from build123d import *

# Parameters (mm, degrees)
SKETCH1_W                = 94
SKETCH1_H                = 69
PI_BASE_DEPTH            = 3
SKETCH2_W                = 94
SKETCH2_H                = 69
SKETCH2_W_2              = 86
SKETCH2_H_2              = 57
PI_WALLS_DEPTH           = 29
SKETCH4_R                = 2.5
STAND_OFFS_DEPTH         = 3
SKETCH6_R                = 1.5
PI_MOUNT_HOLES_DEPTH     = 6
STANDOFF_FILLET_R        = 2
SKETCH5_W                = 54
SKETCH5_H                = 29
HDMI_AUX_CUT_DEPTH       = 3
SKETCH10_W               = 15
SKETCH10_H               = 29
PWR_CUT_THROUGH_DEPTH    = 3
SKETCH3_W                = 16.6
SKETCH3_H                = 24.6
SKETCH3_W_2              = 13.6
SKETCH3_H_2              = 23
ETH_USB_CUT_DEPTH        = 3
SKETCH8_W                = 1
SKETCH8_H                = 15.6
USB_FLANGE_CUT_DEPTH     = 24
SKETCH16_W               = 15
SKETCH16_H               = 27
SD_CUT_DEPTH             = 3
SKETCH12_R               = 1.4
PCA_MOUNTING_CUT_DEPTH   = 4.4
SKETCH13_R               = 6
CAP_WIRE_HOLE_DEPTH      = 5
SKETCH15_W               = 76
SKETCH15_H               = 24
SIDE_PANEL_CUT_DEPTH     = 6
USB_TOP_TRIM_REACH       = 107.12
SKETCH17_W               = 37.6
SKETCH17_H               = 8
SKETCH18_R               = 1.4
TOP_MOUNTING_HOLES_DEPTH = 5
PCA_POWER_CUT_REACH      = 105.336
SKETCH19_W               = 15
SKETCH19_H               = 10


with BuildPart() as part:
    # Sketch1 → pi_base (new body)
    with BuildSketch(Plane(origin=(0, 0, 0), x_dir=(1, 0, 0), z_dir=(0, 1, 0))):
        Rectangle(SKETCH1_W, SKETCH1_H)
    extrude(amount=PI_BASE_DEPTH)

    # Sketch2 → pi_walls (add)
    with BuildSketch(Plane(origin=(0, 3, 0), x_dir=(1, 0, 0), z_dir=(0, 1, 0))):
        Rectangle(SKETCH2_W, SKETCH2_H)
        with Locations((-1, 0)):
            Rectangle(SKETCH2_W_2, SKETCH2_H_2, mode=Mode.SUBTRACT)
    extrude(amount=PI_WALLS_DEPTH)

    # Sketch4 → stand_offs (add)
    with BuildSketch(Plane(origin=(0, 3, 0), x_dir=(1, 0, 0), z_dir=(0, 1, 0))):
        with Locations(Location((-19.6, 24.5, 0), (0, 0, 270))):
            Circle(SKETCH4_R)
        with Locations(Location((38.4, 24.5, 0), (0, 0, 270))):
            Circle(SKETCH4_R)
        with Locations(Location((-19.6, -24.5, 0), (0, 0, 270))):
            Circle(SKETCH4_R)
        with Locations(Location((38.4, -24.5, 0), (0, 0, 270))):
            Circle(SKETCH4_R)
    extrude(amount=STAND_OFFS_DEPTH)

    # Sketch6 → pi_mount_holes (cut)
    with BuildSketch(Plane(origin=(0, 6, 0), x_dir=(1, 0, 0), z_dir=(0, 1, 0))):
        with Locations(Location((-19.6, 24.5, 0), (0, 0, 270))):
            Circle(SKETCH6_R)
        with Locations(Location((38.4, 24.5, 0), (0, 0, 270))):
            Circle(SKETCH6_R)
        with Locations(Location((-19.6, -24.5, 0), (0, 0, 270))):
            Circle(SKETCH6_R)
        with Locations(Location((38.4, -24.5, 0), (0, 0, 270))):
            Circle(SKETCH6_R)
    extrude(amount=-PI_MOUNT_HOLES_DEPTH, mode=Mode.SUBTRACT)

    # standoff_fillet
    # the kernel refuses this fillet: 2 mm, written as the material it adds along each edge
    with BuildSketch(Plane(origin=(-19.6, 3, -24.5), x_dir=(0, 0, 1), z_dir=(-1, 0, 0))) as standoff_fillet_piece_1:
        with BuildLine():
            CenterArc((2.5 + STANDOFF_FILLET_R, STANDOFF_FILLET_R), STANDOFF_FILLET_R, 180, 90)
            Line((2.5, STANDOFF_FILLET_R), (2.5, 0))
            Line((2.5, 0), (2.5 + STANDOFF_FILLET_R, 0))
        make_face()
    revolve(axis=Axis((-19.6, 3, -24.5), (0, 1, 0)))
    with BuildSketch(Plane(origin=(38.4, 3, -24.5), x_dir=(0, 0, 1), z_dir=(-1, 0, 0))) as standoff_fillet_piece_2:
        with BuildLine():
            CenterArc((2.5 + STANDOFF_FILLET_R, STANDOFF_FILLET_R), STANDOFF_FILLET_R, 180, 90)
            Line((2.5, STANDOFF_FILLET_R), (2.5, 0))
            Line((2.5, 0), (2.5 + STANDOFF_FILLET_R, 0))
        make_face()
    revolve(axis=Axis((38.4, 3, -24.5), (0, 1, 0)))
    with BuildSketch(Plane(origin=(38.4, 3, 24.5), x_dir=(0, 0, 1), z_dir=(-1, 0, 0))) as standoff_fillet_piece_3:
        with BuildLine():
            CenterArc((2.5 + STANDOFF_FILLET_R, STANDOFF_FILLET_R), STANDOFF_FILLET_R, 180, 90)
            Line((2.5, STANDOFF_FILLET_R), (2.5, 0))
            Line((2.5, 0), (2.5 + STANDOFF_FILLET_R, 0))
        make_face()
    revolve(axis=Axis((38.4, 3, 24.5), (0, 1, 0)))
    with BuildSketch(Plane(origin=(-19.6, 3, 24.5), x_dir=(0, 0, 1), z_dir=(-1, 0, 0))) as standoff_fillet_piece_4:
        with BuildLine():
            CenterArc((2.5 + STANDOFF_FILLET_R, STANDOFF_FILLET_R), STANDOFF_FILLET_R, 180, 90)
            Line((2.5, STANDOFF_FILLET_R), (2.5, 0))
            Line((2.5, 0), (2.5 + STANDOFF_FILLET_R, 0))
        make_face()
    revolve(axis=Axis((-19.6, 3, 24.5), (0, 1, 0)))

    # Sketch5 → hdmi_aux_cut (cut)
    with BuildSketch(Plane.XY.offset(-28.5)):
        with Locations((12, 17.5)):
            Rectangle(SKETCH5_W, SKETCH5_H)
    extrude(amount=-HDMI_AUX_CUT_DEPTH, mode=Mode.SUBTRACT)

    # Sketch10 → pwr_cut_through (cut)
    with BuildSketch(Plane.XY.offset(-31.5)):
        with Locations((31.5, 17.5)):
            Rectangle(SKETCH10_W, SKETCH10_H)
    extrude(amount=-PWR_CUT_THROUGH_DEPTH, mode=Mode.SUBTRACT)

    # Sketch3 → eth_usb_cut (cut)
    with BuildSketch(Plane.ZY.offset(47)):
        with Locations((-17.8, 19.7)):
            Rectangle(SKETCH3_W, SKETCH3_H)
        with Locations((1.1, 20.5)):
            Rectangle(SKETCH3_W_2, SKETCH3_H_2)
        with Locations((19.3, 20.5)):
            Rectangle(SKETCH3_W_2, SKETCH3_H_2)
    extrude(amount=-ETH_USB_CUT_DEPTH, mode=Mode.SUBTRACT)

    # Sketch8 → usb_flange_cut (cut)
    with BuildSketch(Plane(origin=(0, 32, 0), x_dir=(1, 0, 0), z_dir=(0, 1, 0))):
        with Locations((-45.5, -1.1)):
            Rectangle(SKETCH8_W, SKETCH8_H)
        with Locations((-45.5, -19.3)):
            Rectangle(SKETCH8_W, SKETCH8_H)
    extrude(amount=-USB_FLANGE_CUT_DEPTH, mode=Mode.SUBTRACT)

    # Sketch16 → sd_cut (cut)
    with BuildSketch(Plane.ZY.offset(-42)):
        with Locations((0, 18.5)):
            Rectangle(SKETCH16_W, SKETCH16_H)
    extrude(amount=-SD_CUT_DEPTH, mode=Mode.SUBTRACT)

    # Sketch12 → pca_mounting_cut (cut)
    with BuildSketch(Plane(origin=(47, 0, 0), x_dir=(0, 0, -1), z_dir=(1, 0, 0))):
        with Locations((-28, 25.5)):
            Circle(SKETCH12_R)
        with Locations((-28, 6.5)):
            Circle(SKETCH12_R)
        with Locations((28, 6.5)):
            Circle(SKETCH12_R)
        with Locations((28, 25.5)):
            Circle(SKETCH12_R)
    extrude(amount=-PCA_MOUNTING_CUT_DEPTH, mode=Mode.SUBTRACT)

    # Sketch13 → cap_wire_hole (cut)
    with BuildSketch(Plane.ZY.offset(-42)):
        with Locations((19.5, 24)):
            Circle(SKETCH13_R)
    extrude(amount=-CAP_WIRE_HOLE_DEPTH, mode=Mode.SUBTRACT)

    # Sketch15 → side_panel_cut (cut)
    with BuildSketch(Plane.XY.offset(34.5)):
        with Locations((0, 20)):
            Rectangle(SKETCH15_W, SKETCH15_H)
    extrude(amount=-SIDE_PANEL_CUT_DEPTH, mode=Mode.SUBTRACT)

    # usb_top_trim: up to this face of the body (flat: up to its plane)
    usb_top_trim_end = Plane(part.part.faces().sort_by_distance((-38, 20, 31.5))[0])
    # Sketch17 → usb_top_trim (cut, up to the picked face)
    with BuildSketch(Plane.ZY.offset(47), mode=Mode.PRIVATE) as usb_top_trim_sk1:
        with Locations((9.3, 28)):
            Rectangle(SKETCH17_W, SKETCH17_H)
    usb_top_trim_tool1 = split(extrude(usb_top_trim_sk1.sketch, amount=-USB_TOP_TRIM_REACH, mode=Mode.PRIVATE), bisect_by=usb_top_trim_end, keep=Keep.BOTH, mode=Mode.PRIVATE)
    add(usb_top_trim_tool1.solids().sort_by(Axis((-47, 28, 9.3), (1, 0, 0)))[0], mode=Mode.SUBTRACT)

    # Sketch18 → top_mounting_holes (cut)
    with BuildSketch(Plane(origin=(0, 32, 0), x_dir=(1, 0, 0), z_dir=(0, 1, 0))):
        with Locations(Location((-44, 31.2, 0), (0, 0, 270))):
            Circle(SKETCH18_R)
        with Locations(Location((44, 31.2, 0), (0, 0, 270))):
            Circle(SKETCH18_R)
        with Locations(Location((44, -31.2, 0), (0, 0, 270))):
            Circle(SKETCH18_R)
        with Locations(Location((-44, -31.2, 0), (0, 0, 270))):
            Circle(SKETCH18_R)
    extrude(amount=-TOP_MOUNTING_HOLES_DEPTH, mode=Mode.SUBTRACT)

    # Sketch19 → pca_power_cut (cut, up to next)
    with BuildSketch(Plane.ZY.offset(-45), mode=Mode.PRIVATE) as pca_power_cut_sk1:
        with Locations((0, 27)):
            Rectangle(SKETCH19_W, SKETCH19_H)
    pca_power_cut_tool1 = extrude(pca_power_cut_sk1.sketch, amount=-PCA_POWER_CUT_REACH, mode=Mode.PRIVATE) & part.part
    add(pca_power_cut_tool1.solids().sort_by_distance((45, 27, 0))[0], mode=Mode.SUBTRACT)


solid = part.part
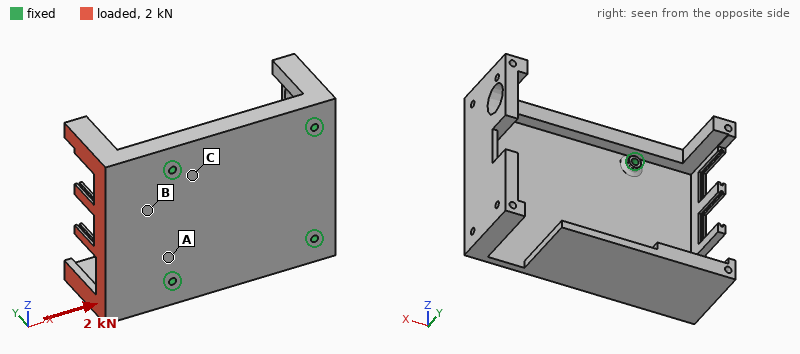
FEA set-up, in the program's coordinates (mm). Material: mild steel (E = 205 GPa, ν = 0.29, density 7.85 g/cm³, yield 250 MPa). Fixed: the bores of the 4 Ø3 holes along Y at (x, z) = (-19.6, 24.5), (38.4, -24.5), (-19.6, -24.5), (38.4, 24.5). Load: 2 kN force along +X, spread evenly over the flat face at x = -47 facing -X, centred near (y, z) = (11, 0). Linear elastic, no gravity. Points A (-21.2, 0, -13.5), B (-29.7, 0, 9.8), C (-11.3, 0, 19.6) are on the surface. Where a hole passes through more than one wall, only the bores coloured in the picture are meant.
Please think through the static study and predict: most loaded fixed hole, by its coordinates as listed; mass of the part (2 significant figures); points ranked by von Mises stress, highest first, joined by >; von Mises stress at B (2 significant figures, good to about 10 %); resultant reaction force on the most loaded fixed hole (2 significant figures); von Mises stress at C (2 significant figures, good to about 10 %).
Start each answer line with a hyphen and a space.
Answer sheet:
- (-19.6, -24.5)
- 340 g
- B > C > A
- 30 MPa
- 820 N
- 18 MPa
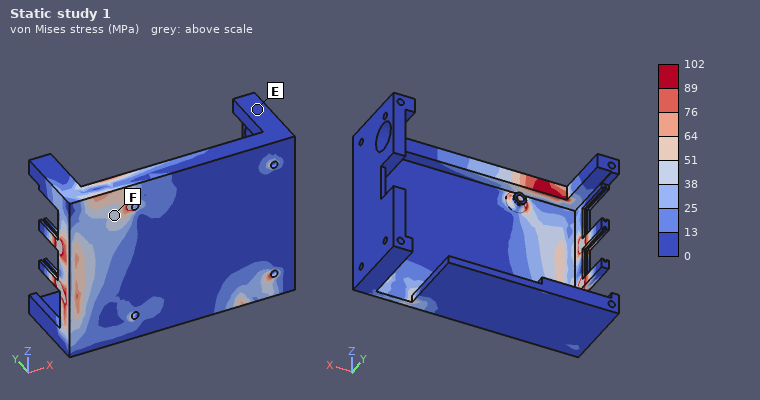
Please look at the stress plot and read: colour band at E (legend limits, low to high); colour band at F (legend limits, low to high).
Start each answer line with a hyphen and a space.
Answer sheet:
- 0 to 13 MPa
- 38 to 51 MPa
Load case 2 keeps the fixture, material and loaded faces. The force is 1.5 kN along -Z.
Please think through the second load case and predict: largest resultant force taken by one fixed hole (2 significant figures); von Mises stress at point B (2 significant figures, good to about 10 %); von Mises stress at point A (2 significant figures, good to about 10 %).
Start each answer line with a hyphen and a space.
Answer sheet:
- 1.1 kN
- 12 MPa
- 13 MPa
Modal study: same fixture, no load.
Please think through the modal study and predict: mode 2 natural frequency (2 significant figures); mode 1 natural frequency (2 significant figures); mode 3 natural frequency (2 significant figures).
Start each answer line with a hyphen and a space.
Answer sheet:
- 2600 Hz
- 2100 Hz
- 2800 Hz
